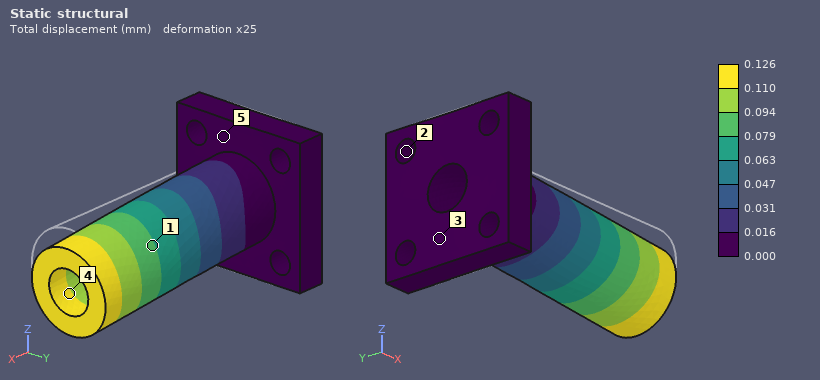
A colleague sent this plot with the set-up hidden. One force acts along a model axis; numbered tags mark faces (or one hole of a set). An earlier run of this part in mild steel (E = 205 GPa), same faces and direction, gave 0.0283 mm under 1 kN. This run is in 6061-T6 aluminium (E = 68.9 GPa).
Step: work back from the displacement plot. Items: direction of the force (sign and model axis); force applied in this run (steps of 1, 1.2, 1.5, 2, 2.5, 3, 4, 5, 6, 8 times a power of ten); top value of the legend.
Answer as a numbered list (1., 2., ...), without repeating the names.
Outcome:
1. -Z
2. 1.5 kN
3. 0.126 mm
